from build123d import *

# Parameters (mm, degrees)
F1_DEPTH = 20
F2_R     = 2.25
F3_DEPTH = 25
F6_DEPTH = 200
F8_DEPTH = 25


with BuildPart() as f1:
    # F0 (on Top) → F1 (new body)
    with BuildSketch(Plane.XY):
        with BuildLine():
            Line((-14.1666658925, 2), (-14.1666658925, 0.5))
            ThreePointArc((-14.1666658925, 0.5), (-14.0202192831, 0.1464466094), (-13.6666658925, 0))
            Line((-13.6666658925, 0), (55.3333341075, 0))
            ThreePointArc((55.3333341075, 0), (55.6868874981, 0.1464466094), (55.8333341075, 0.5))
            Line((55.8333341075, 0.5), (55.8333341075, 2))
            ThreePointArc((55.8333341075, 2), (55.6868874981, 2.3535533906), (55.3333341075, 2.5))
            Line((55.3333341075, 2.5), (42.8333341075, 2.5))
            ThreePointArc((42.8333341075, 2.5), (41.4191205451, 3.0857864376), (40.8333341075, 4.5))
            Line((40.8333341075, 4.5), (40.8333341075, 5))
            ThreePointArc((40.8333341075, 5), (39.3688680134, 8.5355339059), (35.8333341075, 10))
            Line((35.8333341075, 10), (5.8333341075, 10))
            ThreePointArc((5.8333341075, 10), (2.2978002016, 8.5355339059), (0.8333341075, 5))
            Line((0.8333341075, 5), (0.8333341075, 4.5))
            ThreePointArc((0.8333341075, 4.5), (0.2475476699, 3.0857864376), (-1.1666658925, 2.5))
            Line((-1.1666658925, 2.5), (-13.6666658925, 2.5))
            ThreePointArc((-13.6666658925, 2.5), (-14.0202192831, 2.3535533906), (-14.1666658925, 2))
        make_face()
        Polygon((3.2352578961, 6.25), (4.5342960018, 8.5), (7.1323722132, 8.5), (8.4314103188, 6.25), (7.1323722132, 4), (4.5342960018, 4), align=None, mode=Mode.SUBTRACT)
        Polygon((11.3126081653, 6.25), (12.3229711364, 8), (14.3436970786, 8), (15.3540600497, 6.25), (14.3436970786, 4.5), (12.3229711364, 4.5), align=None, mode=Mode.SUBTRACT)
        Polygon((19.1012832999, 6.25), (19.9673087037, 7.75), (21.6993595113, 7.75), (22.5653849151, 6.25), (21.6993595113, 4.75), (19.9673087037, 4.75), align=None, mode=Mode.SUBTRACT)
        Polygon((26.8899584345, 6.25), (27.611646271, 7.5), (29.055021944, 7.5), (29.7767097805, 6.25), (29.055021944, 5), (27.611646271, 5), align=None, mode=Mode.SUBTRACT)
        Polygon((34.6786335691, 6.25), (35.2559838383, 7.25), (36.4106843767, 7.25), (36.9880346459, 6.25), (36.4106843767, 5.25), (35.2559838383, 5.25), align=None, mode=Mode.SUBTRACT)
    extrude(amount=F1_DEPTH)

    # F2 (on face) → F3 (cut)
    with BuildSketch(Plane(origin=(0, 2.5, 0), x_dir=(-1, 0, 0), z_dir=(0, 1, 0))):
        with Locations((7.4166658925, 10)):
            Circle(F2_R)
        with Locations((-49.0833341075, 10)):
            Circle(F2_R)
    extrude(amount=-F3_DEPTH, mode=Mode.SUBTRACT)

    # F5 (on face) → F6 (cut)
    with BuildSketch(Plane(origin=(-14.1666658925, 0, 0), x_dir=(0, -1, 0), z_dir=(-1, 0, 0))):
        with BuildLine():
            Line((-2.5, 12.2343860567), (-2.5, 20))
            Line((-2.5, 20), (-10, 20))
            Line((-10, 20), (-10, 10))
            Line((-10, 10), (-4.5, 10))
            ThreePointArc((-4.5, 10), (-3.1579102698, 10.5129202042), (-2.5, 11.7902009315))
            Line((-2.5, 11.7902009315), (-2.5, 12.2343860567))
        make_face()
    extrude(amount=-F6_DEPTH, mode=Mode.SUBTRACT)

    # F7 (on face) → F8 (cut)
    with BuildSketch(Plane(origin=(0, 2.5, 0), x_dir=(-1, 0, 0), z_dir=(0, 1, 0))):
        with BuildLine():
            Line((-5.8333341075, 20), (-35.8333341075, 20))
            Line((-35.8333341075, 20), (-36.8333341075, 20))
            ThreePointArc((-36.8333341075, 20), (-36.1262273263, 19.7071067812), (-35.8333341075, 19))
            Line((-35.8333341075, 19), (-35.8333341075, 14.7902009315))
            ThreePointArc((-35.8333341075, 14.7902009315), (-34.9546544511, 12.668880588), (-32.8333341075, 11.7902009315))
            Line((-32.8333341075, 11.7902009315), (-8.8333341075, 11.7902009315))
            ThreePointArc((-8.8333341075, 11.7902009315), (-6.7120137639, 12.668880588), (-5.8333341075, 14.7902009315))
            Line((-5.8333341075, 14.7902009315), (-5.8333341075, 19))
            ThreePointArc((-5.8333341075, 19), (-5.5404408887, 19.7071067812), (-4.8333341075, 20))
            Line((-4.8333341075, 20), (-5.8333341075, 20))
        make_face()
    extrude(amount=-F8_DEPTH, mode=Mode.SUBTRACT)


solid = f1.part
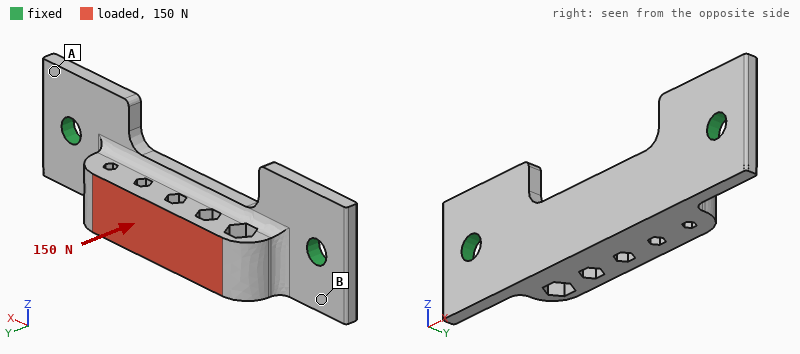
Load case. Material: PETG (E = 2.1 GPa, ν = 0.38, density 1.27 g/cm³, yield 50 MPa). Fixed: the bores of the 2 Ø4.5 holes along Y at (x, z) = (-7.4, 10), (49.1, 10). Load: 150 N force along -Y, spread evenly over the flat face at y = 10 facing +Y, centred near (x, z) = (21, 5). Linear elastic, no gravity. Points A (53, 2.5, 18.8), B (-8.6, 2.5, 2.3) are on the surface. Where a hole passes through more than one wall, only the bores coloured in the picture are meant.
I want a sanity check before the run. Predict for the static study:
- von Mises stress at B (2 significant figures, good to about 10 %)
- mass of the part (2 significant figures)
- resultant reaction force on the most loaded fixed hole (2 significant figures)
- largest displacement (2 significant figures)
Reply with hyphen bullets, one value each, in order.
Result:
- 8.3 MPa
- 6.7 g
- 100 N
- 0.56 mm
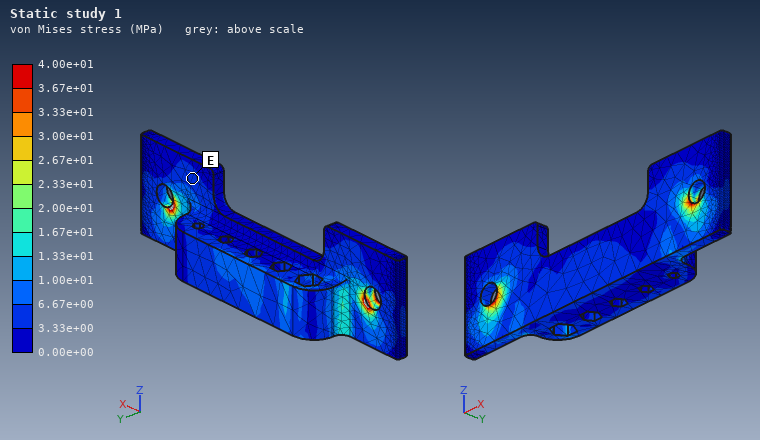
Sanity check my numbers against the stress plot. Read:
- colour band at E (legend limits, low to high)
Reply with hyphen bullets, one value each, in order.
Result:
- 3.33e+00 to 6.67e+00 MPa
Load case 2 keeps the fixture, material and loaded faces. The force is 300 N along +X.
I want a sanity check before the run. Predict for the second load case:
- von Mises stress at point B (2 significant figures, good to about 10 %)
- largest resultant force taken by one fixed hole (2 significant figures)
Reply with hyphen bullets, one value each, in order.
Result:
- 1.8 MPa
- 160 N
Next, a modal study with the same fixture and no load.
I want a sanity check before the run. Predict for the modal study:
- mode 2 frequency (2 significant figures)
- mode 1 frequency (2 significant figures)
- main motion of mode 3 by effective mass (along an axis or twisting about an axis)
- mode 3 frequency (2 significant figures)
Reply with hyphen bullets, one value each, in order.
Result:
- 2400 Hz
- 1400 Hz
- along Z
- 3400 Hz
